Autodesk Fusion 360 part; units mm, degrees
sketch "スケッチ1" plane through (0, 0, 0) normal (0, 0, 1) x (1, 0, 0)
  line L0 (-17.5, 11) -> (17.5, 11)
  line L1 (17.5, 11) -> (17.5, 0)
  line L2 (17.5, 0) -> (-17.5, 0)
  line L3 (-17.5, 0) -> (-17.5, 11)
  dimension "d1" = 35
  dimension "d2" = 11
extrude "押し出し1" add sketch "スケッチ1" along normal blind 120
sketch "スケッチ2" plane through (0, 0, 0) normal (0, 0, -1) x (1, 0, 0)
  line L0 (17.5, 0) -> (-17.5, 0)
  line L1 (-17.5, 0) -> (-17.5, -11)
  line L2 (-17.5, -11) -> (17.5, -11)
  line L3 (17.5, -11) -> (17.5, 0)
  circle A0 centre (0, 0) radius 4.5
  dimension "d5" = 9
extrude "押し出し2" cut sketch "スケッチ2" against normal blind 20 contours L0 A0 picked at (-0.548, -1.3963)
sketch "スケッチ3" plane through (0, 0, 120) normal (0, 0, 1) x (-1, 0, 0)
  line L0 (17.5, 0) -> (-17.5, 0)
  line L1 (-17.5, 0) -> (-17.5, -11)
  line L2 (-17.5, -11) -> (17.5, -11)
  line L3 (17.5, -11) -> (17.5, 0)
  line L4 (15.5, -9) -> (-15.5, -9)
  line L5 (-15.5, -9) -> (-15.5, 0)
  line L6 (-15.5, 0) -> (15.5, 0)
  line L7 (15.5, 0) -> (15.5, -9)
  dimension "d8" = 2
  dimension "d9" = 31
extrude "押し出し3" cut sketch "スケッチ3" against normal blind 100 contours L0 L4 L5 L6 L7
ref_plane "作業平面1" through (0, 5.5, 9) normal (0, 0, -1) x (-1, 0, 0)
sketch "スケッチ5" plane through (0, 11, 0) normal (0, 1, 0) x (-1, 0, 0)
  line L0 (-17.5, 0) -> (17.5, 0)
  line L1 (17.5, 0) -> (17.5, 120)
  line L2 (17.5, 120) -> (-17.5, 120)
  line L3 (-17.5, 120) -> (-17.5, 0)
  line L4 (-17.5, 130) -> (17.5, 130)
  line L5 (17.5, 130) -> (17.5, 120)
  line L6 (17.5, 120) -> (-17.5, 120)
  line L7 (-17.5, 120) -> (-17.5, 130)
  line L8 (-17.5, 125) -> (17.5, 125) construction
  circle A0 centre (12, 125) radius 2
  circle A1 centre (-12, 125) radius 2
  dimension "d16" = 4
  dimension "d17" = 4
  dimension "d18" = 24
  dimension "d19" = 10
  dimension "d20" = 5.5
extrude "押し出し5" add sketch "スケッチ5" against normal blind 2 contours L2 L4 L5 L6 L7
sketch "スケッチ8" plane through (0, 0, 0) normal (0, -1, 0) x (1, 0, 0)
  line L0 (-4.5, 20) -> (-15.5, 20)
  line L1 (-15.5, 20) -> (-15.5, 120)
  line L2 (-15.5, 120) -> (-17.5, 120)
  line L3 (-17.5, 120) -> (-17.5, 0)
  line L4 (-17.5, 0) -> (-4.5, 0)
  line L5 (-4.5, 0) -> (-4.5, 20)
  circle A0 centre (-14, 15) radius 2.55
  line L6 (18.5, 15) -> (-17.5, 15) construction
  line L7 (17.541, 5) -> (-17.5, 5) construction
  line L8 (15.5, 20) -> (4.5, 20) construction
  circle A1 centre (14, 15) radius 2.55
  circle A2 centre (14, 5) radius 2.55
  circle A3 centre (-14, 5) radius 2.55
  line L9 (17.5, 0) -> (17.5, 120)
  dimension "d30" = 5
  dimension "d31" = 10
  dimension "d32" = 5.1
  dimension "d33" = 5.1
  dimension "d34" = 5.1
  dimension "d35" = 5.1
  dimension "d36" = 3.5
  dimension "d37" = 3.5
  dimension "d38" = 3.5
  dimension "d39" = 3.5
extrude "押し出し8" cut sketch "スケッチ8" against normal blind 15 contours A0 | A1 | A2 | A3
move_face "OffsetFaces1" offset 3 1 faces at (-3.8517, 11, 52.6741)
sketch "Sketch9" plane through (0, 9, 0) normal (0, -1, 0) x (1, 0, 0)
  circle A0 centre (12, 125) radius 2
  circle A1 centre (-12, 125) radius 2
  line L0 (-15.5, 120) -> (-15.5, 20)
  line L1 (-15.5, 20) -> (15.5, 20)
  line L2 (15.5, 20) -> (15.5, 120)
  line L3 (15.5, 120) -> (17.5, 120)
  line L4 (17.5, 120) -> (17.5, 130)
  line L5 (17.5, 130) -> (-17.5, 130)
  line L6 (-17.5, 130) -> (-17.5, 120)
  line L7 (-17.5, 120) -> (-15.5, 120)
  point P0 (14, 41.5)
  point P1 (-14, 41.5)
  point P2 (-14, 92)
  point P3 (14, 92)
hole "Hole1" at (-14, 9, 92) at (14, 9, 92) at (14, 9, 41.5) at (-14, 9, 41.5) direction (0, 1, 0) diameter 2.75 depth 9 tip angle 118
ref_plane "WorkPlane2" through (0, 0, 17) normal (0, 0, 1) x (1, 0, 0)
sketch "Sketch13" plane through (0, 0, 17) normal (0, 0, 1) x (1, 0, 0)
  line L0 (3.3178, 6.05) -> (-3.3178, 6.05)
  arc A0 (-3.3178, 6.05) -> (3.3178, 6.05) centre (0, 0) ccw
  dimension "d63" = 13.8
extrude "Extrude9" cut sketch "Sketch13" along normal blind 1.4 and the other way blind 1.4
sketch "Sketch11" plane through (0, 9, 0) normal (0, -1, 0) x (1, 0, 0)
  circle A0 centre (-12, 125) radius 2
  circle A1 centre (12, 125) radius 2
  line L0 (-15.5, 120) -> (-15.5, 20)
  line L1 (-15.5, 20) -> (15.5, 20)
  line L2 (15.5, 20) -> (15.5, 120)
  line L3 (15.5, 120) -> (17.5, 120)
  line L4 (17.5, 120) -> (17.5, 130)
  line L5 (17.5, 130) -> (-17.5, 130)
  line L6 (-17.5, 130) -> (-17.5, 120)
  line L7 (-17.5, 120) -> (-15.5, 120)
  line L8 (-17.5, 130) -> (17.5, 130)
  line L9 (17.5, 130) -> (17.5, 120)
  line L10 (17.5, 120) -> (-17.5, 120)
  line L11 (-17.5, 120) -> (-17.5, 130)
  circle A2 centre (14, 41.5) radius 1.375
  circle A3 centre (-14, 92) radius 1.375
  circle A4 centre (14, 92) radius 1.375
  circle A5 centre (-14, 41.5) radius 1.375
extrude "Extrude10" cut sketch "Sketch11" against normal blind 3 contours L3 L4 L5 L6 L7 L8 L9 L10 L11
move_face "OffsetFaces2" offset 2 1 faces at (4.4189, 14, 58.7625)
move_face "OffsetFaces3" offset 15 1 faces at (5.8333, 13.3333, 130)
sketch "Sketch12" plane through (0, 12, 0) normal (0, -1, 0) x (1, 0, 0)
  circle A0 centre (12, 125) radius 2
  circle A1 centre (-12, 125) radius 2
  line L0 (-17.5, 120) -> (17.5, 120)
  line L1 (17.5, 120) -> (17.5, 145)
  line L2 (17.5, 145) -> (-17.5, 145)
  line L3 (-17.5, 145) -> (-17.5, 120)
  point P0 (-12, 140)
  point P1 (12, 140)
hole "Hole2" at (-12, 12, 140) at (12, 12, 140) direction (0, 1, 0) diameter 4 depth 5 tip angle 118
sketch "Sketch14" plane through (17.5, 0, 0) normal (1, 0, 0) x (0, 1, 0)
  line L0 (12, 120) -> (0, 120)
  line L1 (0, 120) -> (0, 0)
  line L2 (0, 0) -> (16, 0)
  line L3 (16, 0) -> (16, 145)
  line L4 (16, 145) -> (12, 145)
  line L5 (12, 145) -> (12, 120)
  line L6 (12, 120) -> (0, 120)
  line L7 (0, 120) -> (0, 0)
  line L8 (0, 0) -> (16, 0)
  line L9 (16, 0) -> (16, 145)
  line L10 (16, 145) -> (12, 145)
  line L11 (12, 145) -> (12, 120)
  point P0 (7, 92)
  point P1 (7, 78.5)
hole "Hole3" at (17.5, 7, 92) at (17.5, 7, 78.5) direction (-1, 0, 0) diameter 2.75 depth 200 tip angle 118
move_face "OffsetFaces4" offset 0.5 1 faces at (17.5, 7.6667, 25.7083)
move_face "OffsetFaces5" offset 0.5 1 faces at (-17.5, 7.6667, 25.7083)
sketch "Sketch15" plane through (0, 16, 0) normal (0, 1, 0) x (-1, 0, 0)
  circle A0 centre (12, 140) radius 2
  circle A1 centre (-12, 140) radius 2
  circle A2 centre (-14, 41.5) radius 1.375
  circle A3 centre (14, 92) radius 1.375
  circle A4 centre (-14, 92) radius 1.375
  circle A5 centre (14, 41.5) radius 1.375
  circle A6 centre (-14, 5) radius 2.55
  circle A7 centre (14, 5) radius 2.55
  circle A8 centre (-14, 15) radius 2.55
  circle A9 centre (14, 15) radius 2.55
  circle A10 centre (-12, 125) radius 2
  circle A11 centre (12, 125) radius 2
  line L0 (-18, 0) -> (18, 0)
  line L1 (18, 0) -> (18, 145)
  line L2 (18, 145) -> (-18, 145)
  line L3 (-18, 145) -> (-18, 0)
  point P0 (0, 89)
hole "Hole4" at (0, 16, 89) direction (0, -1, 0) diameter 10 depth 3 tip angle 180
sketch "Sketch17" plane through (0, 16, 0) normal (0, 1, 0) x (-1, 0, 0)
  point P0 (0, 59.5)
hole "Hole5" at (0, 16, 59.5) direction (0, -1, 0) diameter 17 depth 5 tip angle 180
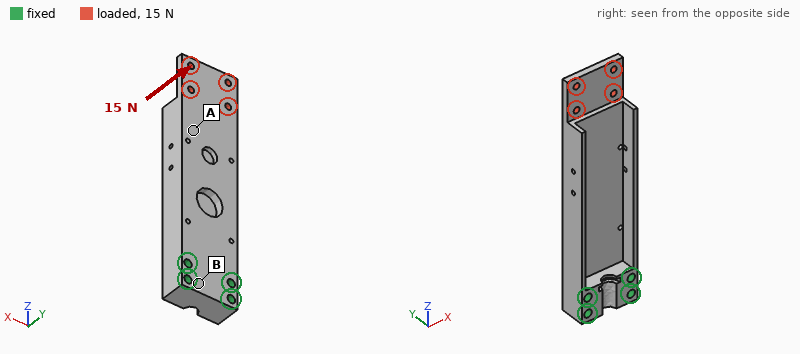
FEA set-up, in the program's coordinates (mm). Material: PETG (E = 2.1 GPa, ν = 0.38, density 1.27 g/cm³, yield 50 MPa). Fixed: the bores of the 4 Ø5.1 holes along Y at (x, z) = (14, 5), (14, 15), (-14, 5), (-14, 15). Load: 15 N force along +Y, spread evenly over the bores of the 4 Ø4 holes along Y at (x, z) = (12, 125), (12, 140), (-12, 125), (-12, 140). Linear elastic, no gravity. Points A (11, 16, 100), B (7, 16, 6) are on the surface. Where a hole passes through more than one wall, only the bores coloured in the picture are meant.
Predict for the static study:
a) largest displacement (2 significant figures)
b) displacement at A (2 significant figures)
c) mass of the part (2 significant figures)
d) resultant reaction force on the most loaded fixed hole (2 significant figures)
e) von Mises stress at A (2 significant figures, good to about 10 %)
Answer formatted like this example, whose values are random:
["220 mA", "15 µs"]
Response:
["1.4 mm", "0.64 mm", "52 g", "19 N", "0.70 MPa"]
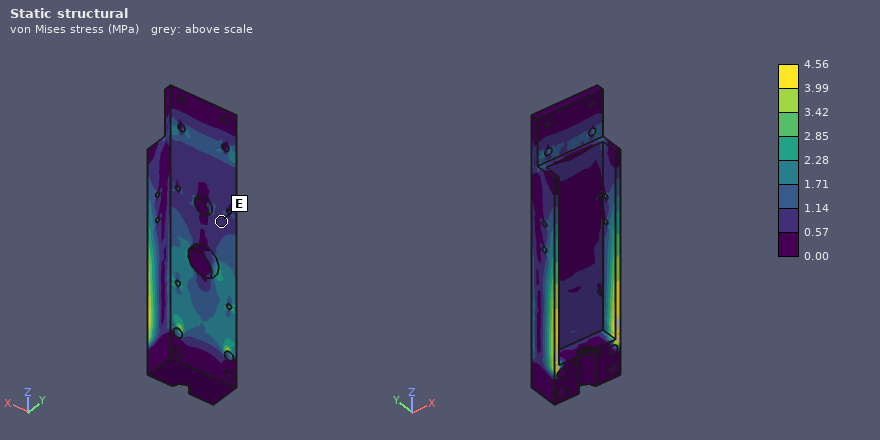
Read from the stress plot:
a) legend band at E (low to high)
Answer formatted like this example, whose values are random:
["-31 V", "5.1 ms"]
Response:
["0.57 to 1.14 MPa"]
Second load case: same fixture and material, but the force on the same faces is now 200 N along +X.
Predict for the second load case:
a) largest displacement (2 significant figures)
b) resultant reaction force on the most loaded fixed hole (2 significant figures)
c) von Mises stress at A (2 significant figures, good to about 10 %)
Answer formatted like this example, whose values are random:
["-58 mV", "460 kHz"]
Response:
["1.8 mm", "760 N", "2.3 MPa"]
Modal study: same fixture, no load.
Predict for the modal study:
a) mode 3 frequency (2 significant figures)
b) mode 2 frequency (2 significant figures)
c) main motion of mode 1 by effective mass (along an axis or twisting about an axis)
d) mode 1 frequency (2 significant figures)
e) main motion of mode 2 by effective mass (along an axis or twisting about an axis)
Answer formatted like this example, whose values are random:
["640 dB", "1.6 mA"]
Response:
["620 Hz", "510 Hz", "along Y", "180 Hz", "along X"]
